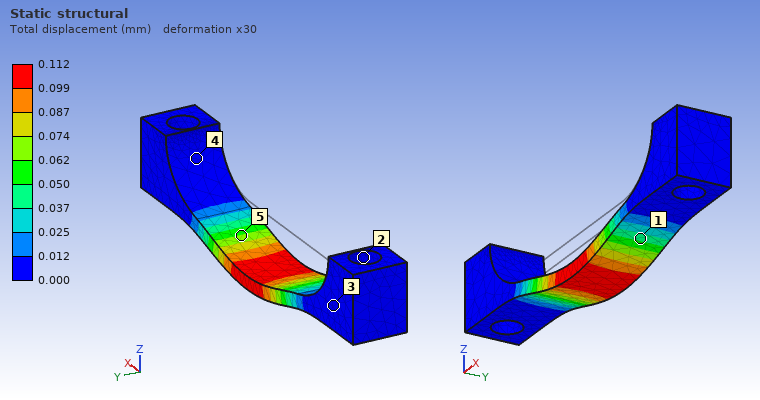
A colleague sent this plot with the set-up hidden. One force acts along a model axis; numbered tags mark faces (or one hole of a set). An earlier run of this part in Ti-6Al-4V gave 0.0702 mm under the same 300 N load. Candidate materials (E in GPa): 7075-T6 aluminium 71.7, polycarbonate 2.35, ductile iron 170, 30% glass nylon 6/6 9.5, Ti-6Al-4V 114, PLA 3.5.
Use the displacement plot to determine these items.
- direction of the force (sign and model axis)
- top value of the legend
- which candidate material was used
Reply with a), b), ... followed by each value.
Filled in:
a) -Z
b) 0.112 mm
c) 7075-T6 aluminium
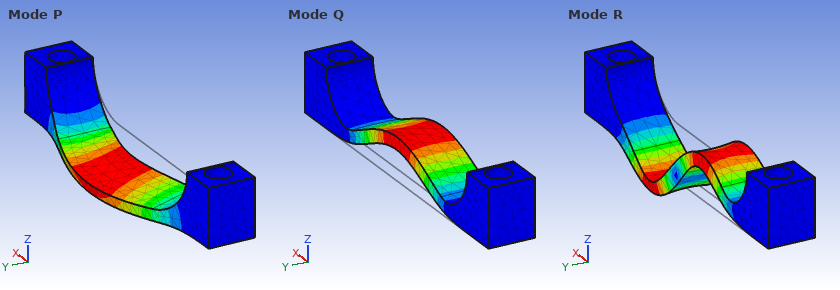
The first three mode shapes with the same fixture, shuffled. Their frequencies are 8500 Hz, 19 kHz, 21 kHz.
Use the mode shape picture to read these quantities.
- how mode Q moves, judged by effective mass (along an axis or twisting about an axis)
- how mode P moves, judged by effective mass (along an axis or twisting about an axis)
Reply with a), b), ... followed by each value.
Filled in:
a) along Z
b) along Y
